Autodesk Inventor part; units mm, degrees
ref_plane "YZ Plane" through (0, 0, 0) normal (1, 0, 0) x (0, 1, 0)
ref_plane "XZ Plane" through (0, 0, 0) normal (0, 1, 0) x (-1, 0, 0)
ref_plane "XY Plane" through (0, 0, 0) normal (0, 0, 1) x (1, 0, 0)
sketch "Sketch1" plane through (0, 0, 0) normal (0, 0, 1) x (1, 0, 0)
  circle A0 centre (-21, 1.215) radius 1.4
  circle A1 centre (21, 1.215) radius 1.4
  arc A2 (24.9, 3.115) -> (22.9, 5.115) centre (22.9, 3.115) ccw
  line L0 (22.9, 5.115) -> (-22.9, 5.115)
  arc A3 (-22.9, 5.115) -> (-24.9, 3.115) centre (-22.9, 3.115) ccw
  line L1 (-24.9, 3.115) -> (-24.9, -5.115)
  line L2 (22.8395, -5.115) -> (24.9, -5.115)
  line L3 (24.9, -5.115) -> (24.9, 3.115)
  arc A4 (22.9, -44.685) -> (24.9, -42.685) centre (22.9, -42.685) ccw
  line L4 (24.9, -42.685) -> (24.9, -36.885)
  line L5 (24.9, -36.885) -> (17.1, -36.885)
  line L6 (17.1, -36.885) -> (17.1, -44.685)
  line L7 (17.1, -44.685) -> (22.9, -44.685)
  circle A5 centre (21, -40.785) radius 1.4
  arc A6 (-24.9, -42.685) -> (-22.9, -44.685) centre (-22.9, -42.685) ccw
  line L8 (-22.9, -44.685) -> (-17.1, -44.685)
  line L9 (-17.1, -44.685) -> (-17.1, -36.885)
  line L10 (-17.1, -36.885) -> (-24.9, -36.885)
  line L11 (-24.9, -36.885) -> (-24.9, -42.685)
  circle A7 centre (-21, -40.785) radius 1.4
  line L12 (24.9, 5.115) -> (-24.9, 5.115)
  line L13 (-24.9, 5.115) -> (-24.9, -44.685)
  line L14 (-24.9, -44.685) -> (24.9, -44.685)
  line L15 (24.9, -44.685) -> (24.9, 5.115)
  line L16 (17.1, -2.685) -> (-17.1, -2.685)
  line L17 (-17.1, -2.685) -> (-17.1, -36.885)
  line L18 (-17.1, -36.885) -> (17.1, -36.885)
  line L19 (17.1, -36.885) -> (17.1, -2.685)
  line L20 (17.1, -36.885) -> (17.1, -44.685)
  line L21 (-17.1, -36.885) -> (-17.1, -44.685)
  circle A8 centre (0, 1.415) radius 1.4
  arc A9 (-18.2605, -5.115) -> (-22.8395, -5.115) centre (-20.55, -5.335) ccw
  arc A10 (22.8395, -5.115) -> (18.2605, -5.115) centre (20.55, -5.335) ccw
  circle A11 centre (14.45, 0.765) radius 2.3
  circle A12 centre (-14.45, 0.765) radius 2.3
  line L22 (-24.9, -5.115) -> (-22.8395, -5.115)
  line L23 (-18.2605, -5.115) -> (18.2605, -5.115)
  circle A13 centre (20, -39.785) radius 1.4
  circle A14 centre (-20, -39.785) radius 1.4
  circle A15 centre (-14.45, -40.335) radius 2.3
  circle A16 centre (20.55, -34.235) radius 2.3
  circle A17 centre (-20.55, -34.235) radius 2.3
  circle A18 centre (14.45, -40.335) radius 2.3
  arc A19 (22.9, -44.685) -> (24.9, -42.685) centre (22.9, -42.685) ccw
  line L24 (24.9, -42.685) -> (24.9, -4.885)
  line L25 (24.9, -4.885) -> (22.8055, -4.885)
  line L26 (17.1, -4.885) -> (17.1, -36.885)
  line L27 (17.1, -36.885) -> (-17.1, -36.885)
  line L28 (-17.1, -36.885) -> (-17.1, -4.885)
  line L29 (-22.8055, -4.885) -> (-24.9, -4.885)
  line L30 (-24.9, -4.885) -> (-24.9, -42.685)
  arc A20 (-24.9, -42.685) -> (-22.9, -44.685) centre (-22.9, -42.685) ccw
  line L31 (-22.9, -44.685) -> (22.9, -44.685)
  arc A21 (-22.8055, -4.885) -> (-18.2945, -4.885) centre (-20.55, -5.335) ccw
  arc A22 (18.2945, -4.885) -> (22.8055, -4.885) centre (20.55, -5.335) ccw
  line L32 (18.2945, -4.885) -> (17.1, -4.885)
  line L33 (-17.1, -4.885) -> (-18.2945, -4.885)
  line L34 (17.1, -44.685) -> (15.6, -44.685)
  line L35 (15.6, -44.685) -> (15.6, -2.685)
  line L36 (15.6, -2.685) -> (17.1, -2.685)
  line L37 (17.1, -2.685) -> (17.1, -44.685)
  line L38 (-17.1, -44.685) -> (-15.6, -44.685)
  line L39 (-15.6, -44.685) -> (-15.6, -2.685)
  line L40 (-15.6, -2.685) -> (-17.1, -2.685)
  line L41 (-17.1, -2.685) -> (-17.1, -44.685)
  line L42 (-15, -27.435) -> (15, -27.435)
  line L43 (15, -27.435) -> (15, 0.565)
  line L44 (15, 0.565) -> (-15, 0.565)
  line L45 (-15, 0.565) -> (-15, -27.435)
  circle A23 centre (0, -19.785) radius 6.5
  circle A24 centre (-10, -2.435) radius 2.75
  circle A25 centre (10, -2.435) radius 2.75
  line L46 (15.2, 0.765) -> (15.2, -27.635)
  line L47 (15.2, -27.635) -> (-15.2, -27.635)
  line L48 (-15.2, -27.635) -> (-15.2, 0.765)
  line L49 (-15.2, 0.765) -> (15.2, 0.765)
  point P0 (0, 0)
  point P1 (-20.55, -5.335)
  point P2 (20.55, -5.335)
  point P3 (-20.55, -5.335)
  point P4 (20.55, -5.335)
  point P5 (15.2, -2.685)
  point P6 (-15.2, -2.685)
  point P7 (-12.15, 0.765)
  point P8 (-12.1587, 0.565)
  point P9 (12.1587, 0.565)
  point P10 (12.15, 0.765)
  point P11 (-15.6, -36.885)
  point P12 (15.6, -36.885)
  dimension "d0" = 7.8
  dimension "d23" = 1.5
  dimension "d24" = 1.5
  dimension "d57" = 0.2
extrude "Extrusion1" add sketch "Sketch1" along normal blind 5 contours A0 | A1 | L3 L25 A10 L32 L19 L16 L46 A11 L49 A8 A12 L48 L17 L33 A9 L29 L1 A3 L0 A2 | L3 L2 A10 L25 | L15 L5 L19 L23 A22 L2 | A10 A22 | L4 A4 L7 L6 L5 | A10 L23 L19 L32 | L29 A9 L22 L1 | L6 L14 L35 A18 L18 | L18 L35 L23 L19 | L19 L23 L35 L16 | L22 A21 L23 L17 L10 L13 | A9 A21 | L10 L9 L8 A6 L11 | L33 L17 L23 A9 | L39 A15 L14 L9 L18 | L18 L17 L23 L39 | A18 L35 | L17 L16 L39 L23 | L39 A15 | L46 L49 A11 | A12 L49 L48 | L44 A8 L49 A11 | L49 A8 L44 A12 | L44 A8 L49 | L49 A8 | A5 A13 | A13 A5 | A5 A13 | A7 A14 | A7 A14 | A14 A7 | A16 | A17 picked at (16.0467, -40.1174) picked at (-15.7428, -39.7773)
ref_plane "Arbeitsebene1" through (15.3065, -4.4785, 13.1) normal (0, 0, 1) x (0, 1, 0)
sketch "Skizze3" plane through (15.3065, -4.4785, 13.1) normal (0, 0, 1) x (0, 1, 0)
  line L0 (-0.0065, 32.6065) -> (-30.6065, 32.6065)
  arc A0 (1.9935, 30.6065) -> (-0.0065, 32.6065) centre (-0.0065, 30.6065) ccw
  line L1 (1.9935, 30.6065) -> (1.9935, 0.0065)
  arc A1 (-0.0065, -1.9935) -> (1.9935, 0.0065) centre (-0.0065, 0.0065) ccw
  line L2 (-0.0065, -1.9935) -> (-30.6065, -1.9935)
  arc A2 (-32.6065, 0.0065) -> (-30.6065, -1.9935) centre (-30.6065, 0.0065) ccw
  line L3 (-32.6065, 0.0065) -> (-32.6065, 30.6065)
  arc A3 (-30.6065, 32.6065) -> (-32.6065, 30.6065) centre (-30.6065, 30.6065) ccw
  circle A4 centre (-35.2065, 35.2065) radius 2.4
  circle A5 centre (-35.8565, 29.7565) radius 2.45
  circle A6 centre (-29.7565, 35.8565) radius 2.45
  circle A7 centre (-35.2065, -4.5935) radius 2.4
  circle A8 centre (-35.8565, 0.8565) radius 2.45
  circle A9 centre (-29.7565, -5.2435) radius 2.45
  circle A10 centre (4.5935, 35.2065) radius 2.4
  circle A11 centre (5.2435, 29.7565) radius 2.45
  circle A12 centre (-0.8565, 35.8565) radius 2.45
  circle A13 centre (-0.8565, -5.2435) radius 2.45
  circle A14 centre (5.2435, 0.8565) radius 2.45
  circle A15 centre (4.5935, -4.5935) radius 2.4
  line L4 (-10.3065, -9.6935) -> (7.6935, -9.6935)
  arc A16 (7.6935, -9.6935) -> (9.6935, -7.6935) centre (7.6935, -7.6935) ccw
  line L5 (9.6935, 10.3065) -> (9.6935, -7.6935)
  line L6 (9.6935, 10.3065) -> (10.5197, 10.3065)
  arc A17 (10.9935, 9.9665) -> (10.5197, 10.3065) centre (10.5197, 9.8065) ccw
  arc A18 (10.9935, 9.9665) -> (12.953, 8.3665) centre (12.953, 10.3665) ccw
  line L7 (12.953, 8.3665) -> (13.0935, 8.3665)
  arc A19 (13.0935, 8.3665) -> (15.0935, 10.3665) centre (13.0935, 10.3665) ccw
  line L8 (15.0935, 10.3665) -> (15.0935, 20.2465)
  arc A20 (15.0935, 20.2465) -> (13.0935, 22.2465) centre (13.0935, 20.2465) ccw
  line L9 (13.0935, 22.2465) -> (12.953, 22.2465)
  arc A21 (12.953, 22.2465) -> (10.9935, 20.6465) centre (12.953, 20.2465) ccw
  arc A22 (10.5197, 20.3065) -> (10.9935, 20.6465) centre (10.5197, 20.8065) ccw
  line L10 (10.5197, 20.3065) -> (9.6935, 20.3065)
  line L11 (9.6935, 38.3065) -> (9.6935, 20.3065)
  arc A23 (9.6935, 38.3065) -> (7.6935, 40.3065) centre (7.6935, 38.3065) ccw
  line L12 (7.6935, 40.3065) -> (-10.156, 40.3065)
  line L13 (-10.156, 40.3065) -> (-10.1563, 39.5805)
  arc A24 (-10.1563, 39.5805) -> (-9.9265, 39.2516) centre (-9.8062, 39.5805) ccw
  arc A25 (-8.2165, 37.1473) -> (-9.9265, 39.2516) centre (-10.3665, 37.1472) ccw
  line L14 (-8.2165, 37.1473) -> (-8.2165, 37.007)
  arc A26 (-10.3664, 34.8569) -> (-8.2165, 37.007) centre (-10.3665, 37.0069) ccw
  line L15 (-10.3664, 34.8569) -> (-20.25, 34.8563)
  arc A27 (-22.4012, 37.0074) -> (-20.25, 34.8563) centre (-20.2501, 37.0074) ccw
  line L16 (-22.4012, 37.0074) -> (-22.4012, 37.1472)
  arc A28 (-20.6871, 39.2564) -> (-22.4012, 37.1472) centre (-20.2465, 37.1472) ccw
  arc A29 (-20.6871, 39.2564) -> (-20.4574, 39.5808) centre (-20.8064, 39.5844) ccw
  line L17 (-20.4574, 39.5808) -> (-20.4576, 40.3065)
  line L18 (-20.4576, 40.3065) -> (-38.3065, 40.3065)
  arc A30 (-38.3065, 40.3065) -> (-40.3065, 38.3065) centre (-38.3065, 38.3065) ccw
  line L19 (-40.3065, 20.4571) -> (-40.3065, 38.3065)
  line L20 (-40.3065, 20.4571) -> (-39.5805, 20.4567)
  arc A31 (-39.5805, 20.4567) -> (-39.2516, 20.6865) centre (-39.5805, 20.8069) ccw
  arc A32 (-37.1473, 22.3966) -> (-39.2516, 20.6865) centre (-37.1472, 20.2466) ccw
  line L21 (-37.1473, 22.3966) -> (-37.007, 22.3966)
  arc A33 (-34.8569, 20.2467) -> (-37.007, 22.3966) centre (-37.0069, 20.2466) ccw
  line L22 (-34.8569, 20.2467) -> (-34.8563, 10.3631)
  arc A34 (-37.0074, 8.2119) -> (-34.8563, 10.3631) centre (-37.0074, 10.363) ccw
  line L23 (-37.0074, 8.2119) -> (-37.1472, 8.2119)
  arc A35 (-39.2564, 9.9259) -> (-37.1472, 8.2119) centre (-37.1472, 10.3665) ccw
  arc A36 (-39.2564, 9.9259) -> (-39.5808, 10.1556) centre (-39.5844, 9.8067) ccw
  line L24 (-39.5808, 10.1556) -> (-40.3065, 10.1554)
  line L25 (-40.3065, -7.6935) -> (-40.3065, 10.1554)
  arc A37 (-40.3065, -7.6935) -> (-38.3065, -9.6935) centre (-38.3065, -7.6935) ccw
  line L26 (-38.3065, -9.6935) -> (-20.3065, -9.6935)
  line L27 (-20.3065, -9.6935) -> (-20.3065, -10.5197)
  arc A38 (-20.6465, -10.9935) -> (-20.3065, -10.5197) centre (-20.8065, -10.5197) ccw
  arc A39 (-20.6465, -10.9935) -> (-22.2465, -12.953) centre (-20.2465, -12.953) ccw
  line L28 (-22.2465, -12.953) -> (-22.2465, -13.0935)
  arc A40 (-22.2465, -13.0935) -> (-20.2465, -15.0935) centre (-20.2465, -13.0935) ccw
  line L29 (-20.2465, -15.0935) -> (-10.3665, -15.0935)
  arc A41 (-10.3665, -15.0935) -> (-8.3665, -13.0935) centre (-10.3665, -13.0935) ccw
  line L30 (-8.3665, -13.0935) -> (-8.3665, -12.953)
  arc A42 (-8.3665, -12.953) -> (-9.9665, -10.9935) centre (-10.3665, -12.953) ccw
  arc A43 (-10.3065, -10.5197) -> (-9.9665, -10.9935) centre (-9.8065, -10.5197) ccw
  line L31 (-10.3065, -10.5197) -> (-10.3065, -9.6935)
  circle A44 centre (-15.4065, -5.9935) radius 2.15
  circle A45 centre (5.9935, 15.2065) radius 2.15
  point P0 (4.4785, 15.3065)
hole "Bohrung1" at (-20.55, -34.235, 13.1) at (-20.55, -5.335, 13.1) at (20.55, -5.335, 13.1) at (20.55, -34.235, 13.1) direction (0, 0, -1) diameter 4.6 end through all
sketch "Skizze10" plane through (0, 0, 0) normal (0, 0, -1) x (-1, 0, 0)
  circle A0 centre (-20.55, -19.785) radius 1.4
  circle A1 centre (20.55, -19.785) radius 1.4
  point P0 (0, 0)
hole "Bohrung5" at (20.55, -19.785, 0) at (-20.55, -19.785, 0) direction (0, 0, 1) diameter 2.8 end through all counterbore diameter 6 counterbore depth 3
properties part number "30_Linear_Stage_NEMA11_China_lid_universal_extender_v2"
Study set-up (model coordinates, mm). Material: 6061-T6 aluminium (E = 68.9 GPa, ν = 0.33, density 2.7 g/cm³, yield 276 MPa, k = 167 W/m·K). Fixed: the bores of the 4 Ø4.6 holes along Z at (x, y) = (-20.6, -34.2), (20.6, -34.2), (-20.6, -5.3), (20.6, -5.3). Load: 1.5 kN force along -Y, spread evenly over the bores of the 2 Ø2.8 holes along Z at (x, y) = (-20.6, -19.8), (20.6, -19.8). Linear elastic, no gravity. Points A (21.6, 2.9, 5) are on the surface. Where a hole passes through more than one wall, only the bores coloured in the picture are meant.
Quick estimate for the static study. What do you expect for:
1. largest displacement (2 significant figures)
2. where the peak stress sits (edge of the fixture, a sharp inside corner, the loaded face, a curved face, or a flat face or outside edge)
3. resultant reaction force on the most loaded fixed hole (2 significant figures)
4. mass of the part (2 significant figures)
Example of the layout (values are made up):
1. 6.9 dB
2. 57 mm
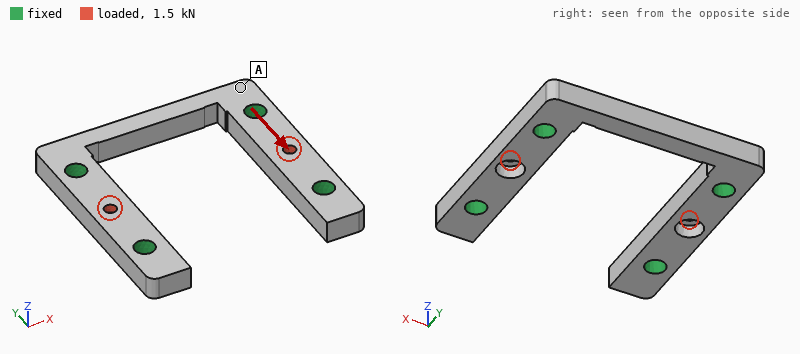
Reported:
1. 3.2 µm
2. the loaded face
3. 380 N
4. 13 g
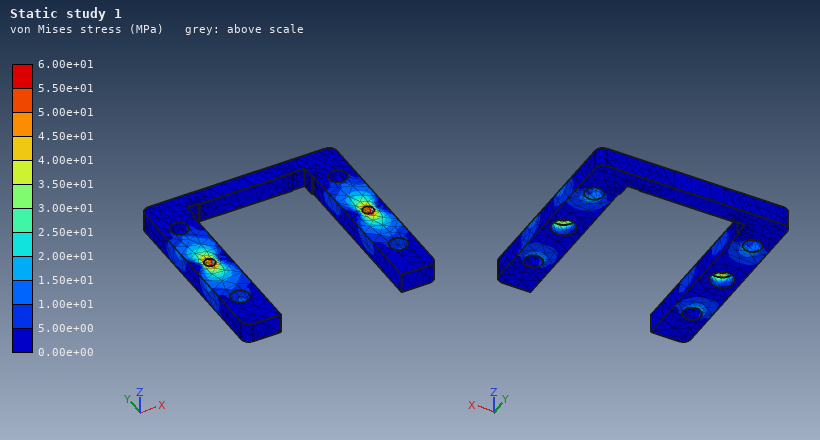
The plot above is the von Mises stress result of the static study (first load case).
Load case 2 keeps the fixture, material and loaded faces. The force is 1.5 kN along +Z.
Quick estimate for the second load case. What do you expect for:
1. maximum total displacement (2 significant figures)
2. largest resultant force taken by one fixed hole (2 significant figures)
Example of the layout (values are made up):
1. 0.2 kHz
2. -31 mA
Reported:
1. 24 µm
2. 400 N
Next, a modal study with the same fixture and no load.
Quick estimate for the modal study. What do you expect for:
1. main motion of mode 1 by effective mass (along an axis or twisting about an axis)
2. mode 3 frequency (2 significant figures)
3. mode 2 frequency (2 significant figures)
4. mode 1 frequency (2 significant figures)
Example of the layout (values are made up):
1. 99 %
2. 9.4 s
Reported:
1. along Z
2. 29 kHz
3. 16 kHz
4. 13 kHz
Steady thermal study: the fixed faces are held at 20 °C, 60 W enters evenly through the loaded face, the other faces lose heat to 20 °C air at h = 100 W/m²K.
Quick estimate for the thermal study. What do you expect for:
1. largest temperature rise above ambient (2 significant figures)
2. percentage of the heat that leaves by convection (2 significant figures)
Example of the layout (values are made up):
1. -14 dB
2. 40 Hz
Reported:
1. 36 K
2. 3.4 %
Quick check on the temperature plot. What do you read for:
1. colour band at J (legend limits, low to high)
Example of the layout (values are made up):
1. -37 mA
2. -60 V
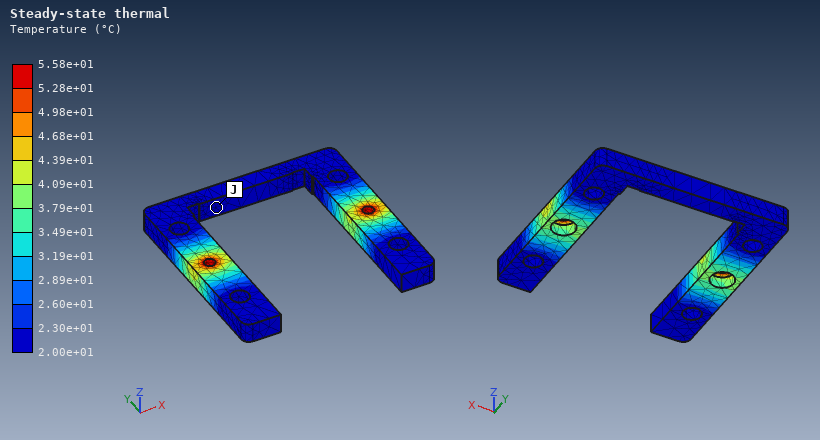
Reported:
1. 2.00e+01 to 2.30e+01 °C
